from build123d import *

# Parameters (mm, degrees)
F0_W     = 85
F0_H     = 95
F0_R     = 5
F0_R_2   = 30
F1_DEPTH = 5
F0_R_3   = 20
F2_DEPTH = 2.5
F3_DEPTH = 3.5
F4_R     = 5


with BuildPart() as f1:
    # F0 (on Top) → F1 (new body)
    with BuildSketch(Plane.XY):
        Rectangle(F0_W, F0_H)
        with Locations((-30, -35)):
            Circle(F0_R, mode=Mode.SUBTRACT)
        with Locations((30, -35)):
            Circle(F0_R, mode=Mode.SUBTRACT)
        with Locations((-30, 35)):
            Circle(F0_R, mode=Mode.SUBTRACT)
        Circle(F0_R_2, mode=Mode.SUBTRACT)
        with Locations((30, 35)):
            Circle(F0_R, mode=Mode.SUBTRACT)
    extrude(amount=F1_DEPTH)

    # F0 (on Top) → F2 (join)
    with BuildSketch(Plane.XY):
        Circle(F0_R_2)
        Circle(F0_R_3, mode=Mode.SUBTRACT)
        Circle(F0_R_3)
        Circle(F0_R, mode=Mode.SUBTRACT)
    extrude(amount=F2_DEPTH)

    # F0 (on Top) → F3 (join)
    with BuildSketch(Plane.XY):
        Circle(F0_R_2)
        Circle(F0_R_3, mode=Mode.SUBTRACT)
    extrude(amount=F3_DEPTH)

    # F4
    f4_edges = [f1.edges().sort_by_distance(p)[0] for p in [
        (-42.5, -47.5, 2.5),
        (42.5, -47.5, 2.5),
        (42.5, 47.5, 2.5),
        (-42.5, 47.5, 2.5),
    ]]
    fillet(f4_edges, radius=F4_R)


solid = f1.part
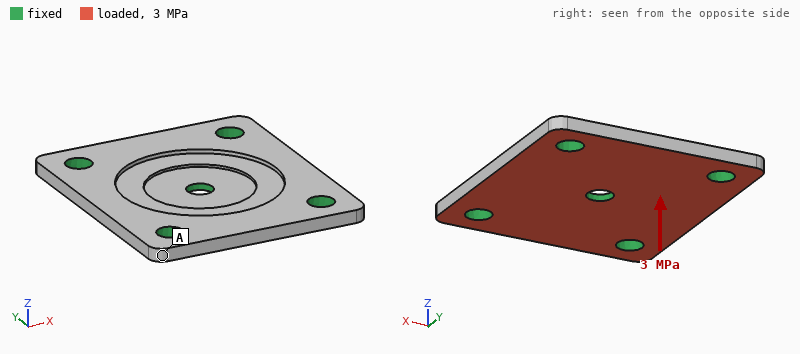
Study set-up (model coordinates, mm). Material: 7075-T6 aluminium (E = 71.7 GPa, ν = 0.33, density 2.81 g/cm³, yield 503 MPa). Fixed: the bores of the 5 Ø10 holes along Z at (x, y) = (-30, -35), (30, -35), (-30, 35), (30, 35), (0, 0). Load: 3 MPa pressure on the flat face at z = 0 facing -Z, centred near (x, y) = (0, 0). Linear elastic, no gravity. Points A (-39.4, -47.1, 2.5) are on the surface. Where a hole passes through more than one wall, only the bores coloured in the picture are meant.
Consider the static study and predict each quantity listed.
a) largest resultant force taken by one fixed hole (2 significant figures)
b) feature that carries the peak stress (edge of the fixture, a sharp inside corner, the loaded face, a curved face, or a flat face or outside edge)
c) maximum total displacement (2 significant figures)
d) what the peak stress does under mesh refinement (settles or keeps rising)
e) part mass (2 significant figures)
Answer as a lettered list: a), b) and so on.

a) 4.8 kN
b) edge of the fixture
c) 0.19 mm
d) keeps rising
e) 93 g
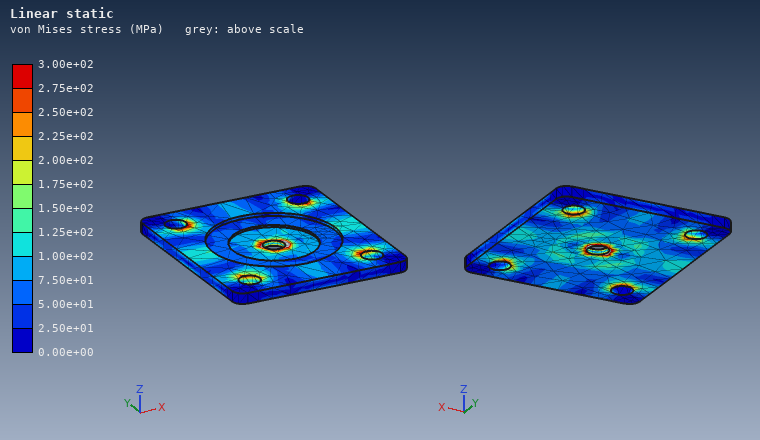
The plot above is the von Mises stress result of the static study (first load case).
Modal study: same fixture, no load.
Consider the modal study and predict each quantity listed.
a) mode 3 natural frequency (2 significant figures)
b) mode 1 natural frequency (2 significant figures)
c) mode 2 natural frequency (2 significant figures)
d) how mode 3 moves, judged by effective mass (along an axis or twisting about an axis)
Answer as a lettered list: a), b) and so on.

a) 8900 Hz
b) 6800 Hz
c) 6900 Hz
d) along Z
